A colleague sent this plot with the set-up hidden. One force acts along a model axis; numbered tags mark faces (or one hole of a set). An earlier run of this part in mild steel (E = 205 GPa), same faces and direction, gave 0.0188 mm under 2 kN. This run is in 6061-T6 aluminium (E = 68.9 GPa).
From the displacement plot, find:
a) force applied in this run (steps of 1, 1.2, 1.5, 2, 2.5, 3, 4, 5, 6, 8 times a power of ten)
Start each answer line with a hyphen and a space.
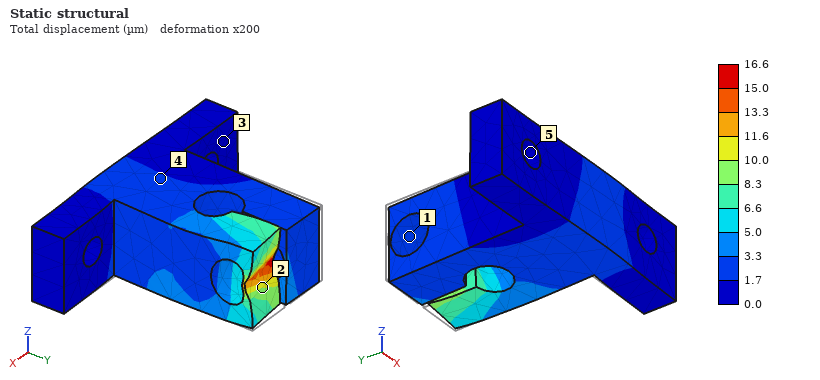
- 600 N
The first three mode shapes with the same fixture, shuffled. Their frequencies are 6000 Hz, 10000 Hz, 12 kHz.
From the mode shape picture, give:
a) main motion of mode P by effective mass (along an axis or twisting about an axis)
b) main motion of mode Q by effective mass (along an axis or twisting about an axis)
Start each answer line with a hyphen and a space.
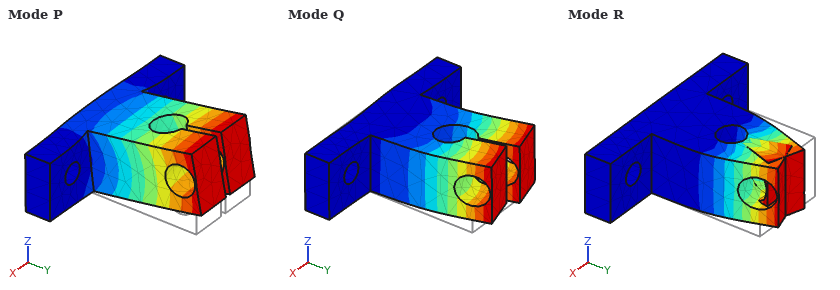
- along Z
- along X
